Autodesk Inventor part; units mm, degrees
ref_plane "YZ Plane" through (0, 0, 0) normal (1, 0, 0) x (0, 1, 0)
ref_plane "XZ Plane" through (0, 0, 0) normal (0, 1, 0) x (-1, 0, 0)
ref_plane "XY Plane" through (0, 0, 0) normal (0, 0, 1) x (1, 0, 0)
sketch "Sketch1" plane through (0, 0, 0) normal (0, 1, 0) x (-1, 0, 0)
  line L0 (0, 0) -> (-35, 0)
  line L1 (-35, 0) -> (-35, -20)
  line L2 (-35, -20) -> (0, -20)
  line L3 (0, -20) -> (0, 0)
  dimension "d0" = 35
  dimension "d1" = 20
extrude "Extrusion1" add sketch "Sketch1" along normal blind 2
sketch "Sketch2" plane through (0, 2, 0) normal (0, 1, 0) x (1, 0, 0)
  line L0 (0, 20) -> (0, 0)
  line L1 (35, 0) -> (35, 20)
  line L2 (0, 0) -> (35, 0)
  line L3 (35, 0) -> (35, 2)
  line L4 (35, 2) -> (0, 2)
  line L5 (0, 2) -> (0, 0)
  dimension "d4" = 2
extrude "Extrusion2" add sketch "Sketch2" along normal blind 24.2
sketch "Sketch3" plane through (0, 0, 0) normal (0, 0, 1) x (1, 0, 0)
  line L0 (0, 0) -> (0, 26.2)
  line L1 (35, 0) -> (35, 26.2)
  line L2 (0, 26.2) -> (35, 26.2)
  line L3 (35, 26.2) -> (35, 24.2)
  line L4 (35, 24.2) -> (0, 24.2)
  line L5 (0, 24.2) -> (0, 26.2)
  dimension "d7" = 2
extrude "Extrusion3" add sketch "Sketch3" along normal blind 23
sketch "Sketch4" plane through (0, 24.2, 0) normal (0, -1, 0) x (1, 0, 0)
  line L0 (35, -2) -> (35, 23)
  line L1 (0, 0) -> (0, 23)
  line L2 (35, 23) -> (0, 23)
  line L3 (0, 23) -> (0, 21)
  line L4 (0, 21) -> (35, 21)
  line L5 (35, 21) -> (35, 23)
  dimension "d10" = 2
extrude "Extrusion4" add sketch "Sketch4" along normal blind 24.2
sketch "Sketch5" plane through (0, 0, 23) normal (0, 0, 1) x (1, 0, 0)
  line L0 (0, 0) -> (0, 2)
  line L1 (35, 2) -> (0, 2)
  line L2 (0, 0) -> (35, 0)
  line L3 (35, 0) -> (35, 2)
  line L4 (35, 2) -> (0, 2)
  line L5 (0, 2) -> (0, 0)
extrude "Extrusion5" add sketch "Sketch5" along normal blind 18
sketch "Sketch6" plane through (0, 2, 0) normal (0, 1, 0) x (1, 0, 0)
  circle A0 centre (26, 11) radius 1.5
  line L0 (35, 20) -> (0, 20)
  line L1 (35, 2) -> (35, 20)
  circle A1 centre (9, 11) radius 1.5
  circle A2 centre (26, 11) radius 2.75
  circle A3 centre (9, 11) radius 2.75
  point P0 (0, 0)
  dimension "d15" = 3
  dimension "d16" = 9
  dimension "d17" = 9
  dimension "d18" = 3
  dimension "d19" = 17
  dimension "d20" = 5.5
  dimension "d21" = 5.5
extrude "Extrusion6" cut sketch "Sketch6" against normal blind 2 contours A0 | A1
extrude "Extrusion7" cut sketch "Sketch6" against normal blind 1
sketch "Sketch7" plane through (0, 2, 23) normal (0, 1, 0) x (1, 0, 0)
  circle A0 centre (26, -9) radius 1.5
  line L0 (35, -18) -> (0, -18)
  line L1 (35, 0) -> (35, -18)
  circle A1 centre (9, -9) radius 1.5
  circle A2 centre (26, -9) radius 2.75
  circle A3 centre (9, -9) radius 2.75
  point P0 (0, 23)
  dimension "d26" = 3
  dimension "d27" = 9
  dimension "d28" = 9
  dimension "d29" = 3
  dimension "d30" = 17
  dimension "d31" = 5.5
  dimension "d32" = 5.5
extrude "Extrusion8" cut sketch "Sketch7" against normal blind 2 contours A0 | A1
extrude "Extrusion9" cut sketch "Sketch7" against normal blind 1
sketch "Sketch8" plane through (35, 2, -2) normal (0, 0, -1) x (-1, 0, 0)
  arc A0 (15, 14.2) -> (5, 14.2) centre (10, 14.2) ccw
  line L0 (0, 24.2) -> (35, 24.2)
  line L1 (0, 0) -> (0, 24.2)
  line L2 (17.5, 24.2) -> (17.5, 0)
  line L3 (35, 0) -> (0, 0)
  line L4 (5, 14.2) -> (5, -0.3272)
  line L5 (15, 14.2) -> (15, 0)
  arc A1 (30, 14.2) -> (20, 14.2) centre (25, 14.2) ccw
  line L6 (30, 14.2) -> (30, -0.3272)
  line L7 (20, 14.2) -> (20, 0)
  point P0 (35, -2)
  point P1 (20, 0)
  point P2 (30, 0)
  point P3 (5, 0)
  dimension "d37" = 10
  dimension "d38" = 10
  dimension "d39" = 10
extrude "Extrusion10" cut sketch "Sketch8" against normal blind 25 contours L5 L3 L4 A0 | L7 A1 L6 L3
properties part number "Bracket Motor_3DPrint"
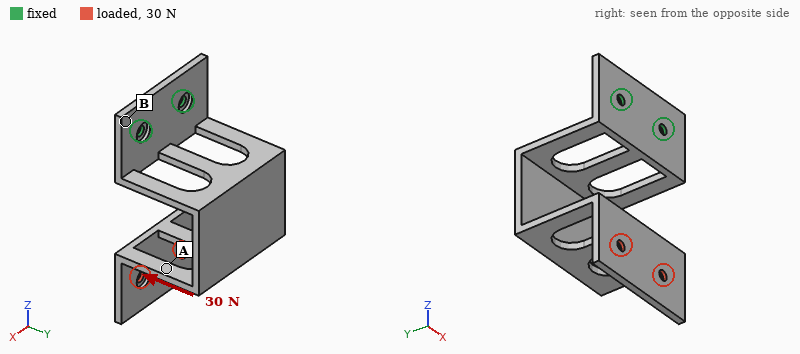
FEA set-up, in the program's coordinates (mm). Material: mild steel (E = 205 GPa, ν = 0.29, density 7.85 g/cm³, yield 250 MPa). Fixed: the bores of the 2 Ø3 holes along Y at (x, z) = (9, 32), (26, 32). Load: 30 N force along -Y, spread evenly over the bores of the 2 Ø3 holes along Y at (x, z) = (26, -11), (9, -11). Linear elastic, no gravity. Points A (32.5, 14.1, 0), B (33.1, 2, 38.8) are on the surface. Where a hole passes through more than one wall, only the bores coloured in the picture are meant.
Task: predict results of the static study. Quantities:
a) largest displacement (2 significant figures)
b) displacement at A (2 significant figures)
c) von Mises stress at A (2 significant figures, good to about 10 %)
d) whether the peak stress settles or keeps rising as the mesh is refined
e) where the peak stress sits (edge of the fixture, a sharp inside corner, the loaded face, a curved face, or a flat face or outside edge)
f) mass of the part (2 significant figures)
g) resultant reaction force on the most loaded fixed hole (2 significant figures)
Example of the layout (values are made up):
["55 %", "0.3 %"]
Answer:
["0.79 mm", "0.36 mm", "28 MPa", "keeps rising", "edge of the fixture", "48 g", "30 N"]
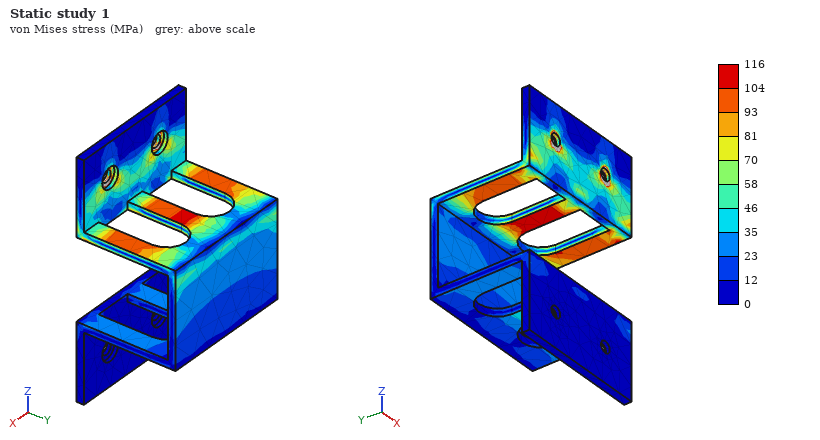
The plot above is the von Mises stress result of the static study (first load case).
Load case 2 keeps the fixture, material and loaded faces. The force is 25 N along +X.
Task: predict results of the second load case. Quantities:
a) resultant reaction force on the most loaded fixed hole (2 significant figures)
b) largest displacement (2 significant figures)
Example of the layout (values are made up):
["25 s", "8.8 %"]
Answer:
["56 N", "0.22 mm"]
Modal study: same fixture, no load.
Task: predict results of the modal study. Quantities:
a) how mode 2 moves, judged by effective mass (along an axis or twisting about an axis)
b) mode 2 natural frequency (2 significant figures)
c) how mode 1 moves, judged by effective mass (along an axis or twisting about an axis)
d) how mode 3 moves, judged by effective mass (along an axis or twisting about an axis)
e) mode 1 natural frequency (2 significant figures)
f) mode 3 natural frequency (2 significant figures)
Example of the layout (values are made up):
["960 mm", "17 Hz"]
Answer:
["along X", "490 Hz", "along Y", "along Z", "260 Hz", "630 Hz"]
